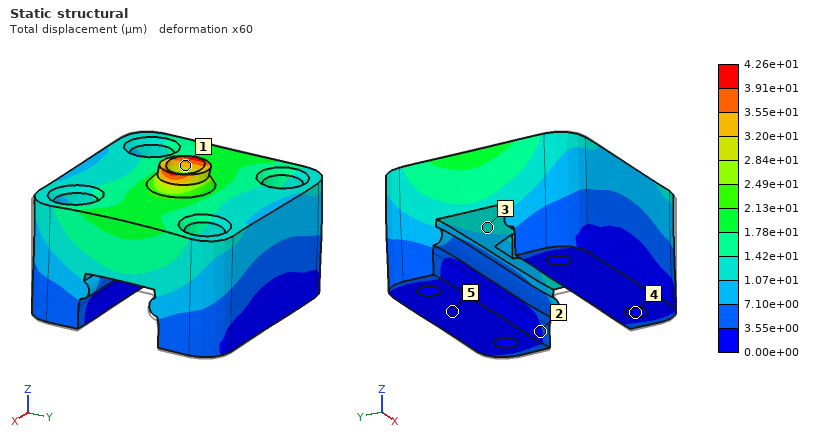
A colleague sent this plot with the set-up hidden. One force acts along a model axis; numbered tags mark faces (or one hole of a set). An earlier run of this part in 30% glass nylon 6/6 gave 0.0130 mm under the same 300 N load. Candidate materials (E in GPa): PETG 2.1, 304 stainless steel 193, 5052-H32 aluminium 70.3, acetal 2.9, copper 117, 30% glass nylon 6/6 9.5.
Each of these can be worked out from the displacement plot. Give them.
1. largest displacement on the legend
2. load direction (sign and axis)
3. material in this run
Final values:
4.26e+01 µm
-X
acetal
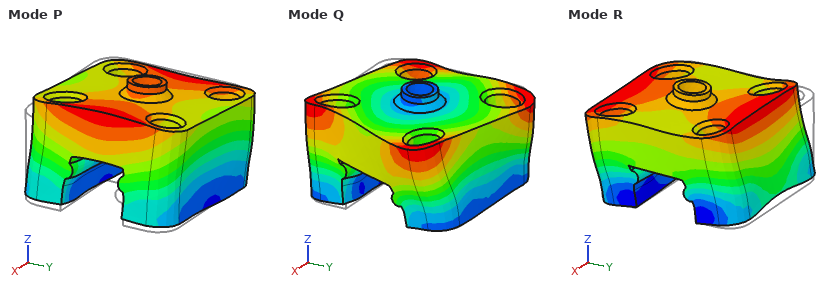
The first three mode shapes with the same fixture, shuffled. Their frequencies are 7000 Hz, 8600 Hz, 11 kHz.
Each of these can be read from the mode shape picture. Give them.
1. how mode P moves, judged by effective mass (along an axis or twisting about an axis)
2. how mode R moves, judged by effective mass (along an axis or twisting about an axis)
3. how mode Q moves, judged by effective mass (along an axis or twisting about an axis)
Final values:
along X
along Y
twisting about Z
